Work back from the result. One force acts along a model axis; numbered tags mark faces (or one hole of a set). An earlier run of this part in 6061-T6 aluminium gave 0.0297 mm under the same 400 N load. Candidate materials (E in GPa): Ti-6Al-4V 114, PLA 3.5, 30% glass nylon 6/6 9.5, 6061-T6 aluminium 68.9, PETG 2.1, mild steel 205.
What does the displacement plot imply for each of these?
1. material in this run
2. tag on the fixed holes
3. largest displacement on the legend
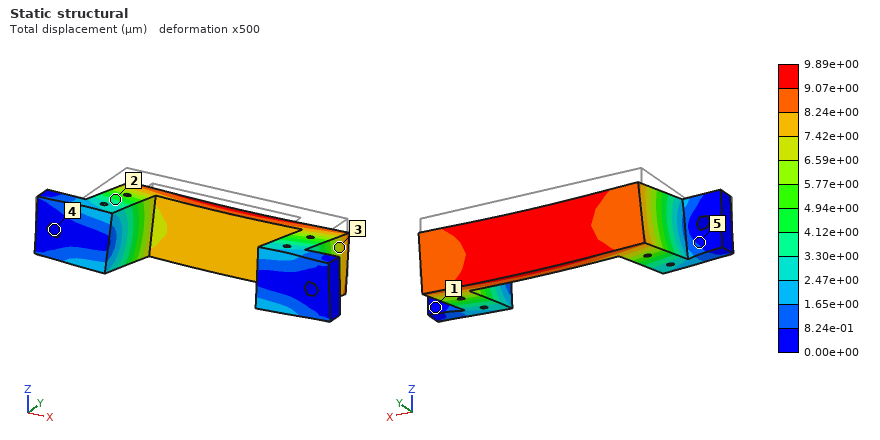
mild steel
4
9.89e+00 µm
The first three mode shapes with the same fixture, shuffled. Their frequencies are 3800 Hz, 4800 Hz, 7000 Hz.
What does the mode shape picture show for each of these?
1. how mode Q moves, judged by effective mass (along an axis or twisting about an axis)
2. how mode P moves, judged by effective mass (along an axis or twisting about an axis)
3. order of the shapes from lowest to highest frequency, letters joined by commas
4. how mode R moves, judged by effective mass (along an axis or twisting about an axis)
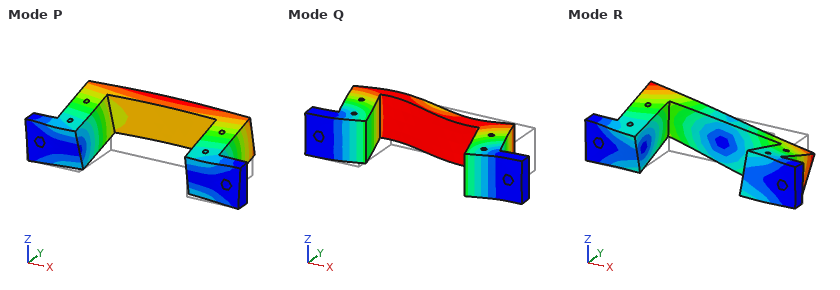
along X
along Z
P, Q, R
twisting about Y
